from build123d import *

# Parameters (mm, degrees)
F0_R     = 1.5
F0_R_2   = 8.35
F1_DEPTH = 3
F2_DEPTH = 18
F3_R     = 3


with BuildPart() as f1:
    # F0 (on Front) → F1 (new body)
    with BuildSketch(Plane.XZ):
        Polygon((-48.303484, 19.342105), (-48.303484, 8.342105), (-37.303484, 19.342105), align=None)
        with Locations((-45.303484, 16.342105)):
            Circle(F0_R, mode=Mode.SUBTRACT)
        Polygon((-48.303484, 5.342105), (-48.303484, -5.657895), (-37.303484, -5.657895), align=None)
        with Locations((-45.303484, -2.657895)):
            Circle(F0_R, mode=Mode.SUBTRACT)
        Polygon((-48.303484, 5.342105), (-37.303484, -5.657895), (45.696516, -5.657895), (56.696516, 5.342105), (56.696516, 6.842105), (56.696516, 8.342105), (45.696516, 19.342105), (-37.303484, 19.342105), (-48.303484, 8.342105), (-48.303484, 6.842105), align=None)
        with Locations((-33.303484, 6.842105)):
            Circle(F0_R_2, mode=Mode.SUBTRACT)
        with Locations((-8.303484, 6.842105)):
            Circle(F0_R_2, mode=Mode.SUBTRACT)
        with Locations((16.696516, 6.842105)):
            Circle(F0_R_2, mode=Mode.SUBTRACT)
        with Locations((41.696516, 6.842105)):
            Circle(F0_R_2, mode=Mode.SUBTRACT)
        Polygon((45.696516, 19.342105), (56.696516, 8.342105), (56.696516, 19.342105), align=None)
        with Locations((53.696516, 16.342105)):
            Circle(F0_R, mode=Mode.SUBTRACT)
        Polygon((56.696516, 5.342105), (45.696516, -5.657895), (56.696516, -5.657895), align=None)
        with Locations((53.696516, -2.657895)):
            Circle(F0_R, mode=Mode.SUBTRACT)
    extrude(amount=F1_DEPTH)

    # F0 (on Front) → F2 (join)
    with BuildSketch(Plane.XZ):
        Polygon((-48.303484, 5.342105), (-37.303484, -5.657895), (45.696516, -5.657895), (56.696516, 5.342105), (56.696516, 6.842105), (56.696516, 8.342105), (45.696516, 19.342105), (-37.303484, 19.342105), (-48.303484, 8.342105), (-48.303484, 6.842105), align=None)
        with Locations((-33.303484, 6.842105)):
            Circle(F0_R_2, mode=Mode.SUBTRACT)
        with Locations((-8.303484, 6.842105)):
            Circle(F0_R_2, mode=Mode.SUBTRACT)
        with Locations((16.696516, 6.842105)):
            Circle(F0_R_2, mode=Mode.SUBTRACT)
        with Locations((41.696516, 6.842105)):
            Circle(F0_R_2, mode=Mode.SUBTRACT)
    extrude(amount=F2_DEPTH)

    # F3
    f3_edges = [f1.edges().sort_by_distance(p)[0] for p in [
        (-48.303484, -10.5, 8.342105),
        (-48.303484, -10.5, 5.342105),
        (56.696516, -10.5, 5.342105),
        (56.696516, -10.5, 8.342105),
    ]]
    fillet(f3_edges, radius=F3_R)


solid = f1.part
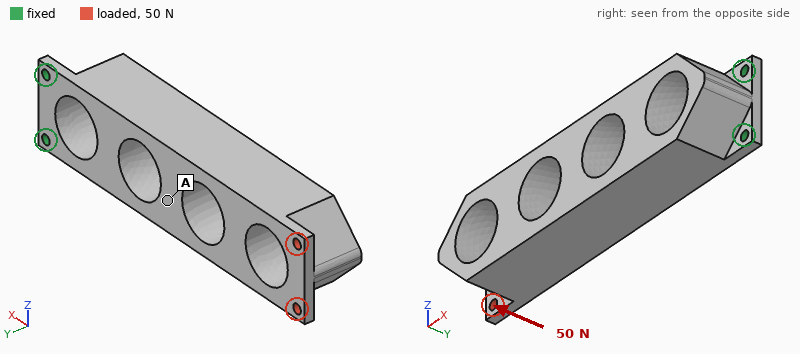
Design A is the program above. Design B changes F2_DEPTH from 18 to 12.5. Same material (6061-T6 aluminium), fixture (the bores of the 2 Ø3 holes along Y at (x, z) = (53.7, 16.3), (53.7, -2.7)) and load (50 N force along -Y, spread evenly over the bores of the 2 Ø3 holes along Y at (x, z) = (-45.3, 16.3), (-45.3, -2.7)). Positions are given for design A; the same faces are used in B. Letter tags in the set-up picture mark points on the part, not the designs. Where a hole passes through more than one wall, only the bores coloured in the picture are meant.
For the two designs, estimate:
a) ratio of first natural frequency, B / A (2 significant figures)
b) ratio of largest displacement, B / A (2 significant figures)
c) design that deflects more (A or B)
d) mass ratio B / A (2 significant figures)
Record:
1.1
1.2
B
0.70
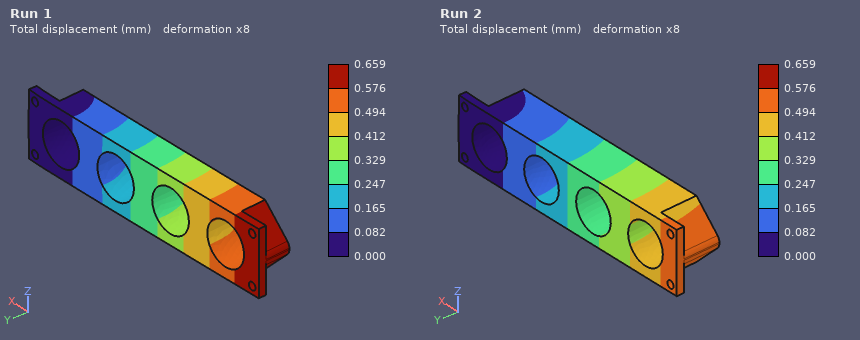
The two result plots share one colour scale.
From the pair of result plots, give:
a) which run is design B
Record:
Run 1
